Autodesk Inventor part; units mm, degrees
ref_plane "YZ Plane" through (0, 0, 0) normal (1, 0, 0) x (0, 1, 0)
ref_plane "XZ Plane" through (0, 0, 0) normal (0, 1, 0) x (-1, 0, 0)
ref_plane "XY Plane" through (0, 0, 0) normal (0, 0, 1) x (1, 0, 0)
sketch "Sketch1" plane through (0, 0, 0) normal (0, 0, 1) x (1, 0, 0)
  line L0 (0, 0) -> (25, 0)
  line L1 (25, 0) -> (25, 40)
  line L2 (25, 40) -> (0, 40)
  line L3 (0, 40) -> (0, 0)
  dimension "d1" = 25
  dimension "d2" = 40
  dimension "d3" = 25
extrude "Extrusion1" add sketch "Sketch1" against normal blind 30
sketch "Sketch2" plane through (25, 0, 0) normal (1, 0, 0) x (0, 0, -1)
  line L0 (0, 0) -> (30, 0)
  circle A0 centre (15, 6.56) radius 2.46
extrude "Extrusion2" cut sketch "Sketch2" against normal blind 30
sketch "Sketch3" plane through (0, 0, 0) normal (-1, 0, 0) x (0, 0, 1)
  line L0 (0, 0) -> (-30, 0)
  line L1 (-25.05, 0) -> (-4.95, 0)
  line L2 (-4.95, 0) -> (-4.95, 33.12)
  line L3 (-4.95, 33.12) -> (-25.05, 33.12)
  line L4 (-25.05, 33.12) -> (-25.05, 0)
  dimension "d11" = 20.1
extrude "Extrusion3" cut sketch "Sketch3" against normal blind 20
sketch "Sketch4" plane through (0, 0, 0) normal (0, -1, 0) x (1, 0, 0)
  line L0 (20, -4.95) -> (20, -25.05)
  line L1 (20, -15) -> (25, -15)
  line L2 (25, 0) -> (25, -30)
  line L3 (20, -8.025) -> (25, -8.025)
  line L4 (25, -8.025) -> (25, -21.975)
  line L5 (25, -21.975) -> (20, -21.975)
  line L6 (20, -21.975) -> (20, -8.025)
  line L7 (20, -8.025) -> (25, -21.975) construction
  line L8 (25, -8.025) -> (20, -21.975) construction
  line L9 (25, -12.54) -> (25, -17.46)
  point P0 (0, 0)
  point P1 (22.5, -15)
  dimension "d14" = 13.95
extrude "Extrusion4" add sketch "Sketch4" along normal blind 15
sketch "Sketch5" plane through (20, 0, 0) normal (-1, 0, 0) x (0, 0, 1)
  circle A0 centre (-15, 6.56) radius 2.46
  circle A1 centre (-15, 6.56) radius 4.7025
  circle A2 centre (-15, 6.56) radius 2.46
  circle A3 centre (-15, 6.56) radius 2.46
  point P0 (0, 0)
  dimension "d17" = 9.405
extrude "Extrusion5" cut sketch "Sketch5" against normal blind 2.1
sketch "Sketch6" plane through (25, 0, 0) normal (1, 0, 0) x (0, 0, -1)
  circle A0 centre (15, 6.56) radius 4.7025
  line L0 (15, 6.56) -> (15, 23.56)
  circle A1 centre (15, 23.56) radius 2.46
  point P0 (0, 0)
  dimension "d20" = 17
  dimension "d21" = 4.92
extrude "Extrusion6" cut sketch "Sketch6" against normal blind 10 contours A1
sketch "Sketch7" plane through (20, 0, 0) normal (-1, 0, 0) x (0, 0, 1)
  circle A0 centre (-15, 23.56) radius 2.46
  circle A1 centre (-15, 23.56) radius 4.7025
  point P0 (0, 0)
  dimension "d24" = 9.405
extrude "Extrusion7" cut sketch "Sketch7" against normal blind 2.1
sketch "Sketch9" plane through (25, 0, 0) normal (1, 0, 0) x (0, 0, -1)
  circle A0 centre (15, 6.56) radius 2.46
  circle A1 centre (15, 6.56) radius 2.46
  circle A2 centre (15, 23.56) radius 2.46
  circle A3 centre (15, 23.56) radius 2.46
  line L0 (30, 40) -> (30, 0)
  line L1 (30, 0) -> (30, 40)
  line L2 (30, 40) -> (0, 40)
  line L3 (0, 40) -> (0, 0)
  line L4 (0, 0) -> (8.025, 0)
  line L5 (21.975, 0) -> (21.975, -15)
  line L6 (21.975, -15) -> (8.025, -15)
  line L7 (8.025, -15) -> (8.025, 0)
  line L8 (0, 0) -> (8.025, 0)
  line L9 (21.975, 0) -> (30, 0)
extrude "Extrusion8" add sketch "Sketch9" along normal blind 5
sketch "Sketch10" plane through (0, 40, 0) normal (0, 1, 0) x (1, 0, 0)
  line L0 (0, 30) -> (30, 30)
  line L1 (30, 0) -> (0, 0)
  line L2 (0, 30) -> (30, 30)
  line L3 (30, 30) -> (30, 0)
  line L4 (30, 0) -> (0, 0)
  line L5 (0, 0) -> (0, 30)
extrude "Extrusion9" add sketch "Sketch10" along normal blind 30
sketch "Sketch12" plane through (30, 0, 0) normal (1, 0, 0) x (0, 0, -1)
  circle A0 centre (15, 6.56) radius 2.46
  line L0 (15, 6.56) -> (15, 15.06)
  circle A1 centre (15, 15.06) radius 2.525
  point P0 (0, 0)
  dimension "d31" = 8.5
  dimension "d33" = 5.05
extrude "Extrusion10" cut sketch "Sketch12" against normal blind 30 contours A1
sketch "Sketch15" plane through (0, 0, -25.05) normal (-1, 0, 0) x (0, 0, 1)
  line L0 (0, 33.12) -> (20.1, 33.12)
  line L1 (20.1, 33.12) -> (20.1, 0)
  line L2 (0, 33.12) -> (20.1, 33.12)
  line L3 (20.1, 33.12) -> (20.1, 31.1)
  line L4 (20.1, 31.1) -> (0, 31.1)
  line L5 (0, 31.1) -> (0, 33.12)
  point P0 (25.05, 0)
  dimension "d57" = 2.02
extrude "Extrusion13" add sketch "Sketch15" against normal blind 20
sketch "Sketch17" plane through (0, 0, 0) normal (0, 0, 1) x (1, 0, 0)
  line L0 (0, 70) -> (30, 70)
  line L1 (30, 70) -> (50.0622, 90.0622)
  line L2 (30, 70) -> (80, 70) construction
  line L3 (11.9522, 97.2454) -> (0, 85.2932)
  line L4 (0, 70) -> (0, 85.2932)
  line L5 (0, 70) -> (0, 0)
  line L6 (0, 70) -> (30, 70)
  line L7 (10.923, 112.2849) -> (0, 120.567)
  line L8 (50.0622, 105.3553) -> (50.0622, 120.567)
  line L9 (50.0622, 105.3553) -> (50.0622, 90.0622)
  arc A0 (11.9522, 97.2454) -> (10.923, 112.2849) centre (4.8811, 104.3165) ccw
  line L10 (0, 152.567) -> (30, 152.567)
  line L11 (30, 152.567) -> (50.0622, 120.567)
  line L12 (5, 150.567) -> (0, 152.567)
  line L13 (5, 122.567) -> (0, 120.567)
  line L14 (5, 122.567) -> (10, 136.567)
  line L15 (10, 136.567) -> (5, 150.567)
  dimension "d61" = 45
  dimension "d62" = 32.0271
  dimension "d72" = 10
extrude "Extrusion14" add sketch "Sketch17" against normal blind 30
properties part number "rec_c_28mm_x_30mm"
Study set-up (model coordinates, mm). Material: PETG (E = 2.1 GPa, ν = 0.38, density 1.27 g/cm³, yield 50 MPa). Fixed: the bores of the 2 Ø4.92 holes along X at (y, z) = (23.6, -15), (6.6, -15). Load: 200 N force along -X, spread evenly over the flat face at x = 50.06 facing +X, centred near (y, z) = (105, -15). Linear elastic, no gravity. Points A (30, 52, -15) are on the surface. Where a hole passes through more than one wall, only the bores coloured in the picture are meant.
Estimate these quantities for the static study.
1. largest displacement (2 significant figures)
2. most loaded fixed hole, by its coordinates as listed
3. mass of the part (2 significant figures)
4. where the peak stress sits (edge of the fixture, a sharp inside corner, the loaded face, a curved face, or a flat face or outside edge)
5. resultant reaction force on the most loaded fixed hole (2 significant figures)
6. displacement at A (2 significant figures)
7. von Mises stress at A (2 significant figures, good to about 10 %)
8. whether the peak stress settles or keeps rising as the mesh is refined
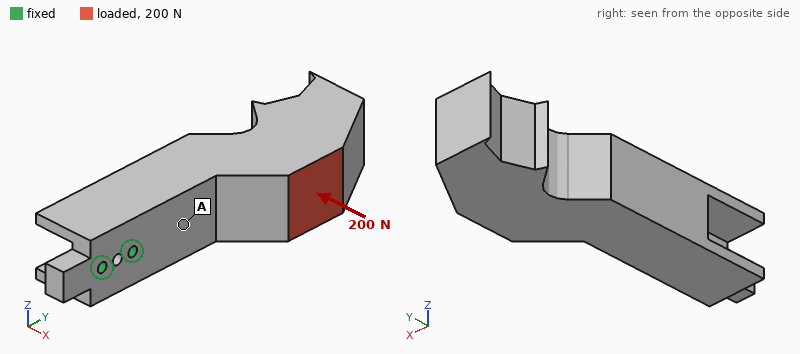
2.0 mm
(23.6, -15)
180 g
edge of the fixture
840 N
0.40 mm
2.3 MPa
keeps rising
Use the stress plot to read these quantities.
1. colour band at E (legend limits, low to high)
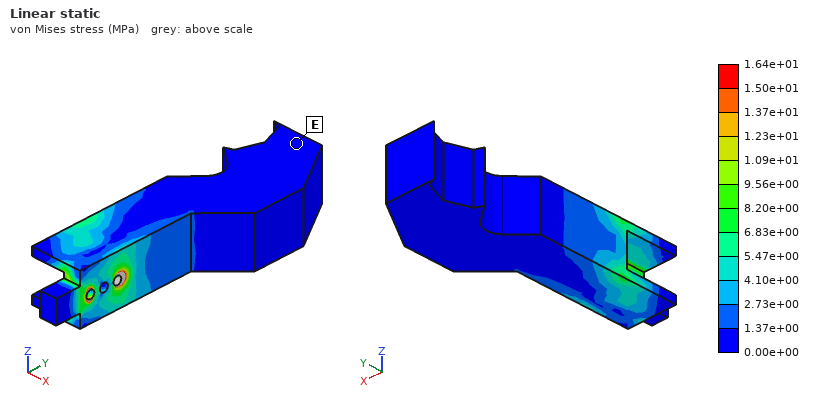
0.00e+00 to 1.37e+00 MPa
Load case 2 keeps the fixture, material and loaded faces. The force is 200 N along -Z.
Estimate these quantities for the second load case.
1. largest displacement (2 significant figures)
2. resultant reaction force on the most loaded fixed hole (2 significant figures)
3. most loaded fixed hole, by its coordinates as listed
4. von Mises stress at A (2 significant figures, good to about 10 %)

1.7 mm
910 N
(23.6, -15)
3.6 MPa
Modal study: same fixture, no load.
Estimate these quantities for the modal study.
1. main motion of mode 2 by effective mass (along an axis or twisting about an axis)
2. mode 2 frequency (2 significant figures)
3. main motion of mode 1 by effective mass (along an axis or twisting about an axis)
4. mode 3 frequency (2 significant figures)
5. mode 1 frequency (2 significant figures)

along Z
190 Hz
along X
580 Hz
170 Hz
